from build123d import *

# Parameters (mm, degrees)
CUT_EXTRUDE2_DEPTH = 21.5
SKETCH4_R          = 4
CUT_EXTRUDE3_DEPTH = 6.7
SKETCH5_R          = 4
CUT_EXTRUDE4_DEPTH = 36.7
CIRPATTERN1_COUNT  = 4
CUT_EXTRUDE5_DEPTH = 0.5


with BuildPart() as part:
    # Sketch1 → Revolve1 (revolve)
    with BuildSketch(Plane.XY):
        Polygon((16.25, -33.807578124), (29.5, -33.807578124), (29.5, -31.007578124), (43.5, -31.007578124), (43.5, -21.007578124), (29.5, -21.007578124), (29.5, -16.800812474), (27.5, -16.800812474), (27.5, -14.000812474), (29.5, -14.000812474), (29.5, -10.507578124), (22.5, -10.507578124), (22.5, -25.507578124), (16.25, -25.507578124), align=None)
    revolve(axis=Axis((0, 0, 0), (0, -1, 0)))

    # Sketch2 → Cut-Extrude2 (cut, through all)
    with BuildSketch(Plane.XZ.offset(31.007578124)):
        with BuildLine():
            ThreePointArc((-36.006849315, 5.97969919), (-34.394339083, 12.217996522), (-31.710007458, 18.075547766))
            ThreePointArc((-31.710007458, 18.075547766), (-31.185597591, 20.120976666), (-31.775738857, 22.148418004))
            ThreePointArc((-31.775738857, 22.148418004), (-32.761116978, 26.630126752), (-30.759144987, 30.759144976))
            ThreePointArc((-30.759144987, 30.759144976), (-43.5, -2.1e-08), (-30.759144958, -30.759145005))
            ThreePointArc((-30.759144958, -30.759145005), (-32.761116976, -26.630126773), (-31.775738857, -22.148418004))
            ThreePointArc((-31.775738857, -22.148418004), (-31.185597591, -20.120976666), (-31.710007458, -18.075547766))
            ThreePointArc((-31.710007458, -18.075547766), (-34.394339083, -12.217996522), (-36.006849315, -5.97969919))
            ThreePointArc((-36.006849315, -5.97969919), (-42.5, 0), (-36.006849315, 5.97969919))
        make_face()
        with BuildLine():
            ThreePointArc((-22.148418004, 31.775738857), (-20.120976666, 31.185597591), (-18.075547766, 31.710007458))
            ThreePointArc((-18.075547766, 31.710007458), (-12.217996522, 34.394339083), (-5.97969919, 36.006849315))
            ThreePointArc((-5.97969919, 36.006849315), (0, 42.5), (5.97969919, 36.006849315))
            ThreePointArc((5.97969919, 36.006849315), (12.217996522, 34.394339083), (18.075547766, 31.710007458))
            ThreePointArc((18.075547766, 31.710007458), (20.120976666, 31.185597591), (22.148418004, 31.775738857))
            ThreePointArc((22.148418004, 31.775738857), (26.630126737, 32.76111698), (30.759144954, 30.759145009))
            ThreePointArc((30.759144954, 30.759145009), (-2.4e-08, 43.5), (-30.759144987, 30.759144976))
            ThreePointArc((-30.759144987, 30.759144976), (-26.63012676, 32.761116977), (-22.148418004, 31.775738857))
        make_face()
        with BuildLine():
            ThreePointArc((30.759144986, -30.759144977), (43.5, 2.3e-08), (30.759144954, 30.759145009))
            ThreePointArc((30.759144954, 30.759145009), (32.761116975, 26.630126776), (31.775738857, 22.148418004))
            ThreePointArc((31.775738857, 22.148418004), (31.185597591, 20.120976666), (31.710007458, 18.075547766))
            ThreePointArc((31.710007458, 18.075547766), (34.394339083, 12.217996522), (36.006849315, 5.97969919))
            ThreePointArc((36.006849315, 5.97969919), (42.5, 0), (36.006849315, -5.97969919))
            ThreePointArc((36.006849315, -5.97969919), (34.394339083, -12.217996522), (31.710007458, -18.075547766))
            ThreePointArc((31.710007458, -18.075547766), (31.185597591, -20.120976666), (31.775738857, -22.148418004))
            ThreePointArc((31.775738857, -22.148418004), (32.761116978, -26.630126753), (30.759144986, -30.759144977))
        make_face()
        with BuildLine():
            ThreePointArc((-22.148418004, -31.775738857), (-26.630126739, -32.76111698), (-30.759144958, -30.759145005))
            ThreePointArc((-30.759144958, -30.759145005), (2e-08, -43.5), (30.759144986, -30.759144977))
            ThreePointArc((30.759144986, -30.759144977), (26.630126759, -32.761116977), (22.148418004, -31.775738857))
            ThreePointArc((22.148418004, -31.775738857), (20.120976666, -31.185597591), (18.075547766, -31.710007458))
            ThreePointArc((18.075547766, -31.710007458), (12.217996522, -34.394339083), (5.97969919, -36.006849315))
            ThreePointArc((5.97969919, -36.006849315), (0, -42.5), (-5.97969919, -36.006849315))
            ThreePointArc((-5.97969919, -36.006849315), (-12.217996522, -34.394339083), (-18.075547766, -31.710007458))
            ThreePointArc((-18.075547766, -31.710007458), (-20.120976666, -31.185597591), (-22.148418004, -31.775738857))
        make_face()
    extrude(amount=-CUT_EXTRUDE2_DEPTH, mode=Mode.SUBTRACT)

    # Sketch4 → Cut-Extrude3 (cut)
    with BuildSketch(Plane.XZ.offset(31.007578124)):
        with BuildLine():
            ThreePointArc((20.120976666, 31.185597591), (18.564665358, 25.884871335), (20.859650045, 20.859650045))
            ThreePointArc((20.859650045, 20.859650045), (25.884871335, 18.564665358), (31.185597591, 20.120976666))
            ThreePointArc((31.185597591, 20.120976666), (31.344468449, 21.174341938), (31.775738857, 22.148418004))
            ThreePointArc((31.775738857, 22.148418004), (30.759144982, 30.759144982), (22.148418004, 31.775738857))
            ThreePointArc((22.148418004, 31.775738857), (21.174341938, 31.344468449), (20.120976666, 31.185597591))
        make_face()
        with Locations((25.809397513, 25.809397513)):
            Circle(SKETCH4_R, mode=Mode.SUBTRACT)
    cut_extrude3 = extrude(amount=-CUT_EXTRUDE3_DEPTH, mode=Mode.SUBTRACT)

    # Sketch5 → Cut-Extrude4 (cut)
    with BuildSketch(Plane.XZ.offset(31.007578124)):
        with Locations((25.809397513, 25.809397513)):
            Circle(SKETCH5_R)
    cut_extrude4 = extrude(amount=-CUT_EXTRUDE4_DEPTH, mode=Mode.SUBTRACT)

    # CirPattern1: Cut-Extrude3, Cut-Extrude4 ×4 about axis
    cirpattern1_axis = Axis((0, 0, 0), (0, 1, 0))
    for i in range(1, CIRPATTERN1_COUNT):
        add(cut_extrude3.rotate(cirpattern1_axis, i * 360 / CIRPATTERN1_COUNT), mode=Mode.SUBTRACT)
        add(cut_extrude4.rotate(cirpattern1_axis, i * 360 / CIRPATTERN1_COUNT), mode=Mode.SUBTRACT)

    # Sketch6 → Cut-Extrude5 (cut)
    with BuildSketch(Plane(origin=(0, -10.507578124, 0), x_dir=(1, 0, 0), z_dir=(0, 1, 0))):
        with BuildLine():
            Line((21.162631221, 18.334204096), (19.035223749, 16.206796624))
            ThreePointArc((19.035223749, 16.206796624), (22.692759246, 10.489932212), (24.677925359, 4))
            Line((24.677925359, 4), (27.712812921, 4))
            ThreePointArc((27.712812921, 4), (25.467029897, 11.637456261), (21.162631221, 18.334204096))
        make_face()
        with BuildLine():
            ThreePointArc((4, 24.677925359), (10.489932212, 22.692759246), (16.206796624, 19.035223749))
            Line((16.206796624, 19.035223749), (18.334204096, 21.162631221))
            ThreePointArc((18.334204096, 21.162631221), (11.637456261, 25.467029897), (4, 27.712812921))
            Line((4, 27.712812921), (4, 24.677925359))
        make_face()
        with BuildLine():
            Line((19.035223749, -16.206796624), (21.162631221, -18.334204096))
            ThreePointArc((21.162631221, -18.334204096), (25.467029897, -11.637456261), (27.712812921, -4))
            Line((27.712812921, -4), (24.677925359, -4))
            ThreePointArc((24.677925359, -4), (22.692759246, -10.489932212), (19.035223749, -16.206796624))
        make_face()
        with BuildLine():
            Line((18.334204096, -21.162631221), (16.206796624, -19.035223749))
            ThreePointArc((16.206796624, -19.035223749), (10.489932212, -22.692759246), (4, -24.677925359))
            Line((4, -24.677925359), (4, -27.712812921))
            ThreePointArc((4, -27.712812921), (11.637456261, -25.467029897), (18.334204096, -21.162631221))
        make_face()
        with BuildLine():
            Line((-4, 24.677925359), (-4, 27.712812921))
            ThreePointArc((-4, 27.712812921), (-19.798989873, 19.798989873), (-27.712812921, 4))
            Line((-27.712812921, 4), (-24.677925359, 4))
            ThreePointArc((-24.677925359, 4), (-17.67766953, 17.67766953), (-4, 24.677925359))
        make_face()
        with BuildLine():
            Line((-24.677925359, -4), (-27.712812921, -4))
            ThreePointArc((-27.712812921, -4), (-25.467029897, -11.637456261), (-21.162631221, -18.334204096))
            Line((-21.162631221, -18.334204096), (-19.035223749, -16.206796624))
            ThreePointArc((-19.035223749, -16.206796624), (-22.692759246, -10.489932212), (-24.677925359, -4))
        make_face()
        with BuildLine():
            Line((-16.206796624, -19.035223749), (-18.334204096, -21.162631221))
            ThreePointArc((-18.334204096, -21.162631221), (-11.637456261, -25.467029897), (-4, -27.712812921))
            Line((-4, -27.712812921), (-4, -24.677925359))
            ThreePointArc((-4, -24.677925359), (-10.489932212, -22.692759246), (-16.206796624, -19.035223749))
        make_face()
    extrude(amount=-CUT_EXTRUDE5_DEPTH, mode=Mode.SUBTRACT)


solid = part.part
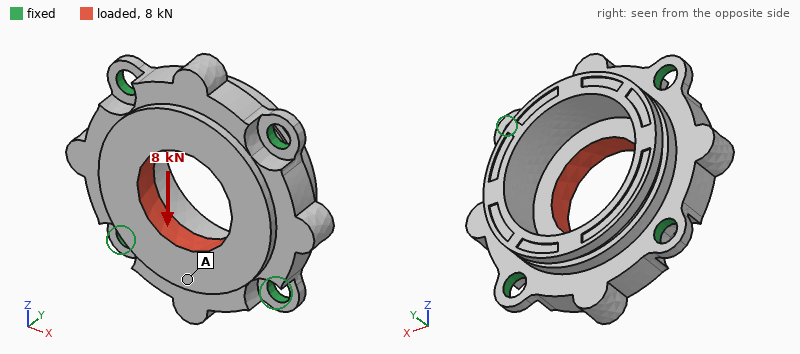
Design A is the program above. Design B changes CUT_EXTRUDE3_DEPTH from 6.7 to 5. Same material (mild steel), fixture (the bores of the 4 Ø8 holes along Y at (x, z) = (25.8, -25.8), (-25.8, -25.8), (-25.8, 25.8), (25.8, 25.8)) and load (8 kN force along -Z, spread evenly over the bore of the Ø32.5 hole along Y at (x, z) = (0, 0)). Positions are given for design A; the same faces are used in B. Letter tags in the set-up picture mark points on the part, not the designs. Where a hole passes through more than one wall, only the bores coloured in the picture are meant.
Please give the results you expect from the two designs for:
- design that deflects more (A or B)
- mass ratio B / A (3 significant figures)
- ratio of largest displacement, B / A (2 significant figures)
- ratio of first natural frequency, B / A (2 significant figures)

A
1.02
0.84
1.1
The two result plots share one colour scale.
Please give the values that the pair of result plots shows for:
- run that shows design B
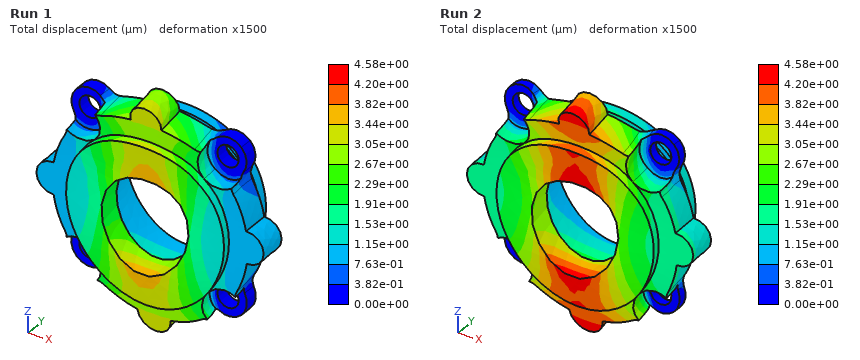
Run 1
